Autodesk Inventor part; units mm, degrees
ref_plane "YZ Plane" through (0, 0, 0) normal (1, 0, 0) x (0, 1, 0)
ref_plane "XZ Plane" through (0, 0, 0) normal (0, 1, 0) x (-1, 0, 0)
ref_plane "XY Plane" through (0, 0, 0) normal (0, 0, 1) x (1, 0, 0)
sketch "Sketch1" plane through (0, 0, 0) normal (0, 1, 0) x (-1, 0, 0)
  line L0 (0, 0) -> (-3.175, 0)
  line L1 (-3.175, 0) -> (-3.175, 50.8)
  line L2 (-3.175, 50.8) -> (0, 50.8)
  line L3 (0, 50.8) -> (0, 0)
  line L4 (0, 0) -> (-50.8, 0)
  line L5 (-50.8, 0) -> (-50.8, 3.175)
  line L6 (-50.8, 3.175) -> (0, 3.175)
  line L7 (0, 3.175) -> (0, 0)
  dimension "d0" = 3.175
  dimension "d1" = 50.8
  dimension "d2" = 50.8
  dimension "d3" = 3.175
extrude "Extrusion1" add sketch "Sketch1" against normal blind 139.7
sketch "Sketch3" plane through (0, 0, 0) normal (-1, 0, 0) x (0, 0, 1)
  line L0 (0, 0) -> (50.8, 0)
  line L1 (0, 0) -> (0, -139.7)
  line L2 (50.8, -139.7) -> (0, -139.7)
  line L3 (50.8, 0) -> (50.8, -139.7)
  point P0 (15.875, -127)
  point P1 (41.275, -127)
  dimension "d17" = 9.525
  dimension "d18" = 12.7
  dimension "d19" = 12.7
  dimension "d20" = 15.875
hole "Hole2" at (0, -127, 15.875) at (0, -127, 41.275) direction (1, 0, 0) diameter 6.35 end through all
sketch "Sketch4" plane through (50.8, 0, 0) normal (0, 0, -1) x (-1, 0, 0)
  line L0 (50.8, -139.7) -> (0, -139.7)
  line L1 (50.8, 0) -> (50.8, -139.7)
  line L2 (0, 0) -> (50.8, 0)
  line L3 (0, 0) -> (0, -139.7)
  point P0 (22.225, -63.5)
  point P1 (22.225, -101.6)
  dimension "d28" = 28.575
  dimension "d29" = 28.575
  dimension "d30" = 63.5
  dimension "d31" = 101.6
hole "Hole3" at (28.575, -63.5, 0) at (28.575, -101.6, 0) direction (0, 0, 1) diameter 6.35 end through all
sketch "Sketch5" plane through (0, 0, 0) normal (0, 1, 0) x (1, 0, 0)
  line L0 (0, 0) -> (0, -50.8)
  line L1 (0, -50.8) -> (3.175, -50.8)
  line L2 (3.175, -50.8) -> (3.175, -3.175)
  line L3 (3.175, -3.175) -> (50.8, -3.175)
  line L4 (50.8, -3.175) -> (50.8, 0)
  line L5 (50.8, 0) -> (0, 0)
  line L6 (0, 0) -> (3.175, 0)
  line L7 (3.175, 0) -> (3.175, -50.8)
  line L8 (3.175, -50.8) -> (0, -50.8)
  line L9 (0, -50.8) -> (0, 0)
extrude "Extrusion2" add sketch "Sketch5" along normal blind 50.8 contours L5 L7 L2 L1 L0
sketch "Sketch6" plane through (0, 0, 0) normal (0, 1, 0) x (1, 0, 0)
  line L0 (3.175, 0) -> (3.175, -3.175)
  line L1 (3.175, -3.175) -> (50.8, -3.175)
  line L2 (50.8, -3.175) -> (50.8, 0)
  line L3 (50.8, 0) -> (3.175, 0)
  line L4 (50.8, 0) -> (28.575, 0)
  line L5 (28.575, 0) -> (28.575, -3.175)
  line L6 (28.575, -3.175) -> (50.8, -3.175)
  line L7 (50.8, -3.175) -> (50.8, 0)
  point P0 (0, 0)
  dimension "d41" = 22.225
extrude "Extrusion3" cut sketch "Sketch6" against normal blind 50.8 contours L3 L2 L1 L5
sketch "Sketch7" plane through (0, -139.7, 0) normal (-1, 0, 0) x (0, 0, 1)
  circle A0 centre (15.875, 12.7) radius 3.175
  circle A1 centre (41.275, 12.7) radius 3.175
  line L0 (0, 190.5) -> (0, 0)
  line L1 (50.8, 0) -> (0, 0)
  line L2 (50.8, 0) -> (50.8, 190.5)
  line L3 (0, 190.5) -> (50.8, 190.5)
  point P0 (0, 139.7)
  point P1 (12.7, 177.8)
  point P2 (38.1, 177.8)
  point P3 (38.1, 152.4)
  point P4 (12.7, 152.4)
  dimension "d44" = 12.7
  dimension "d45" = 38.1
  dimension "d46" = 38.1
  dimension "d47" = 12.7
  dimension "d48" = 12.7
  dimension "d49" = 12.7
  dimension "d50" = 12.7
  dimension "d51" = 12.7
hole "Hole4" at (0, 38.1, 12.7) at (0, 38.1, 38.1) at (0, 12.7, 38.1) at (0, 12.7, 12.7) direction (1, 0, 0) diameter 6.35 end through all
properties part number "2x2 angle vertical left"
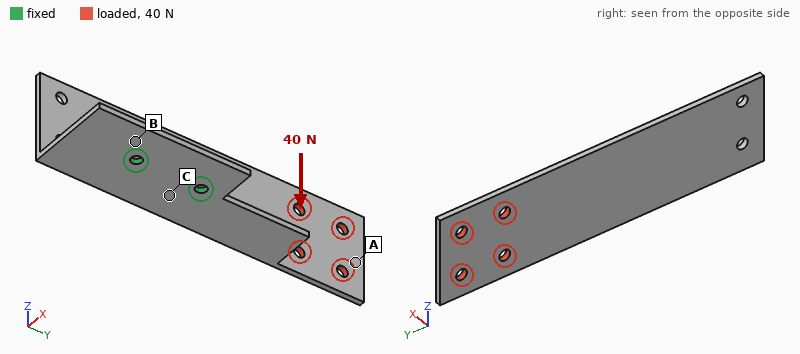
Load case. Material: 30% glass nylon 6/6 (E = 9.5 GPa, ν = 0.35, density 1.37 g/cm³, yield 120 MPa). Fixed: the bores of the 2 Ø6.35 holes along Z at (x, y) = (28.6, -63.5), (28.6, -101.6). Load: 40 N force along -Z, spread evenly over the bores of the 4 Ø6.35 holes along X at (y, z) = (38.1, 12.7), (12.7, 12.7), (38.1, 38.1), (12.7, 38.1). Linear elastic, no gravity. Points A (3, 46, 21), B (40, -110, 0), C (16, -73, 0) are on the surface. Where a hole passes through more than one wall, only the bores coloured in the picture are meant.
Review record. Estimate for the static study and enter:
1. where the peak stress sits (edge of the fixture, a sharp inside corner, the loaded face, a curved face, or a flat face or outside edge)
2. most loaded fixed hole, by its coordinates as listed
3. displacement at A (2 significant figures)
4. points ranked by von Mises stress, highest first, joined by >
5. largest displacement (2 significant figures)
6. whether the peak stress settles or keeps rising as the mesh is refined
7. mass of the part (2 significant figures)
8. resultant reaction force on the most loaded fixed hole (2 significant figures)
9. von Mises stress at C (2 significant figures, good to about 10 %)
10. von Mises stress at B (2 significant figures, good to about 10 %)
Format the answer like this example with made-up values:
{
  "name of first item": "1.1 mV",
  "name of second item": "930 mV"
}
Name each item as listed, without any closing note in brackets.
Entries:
{
  "where the peak stress sits": "edge of the fixture",
  "most loaded fixed hole, by its coordinates as listed": "(28.6, -63.5)",
  "displacement at A": "1.6 mm",
  "points ranked by von Mises stress, highest first, joined by >": "C > B > A",
  "largest displacement": "2.0 mm",
  "whether the peak stress settles or keeps rising as the mesh is refined": "keeps rising",
  "mass of the part": "65 g",
  "resultant reaction force on the most loaded fixed hole": "110 N",
  "von Mises stress at C": "14 MPa",
  "von Mises stress at B": "5.7 MPa"
}
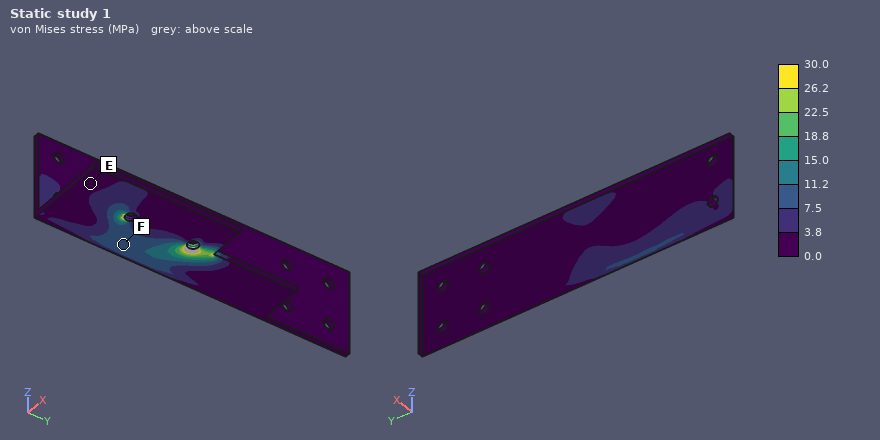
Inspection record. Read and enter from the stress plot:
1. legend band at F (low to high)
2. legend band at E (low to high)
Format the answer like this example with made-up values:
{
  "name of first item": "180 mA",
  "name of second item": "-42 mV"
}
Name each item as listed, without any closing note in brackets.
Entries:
{
  "legend band at F": "7.5 to 11.2 MPa",
  "legend band at E": "0.0 to 3.8 MPa"
}
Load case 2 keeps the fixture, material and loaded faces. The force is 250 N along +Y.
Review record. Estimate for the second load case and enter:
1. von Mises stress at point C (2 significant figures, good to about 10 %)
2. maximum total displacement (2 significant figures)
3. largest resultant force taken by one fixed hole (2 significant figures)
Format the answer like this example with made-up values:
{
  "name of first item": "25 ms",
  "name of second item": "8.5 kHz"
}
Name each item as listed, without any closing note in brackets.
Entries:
{
  "von Mises stress at point C": "12 MPa",
  "maximum total displacement": "2.3 mm",
  "largest resultant force taken by one fixed hole": "240 N"
}
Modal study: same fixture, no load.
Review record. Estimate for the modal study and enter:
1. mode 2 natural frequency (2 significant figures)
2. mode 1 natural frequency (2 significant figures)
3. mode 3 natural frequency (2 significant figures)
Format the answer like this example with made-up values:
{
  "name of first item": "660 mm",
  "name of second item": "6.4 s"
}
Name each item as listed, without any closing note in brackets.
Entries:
{
  "mode 2 natural frequency": "240 Hz",
  "mode 1 natural frequency": "170 Hz",
  "mode 3 natural frequency": "310 Hz"
}
